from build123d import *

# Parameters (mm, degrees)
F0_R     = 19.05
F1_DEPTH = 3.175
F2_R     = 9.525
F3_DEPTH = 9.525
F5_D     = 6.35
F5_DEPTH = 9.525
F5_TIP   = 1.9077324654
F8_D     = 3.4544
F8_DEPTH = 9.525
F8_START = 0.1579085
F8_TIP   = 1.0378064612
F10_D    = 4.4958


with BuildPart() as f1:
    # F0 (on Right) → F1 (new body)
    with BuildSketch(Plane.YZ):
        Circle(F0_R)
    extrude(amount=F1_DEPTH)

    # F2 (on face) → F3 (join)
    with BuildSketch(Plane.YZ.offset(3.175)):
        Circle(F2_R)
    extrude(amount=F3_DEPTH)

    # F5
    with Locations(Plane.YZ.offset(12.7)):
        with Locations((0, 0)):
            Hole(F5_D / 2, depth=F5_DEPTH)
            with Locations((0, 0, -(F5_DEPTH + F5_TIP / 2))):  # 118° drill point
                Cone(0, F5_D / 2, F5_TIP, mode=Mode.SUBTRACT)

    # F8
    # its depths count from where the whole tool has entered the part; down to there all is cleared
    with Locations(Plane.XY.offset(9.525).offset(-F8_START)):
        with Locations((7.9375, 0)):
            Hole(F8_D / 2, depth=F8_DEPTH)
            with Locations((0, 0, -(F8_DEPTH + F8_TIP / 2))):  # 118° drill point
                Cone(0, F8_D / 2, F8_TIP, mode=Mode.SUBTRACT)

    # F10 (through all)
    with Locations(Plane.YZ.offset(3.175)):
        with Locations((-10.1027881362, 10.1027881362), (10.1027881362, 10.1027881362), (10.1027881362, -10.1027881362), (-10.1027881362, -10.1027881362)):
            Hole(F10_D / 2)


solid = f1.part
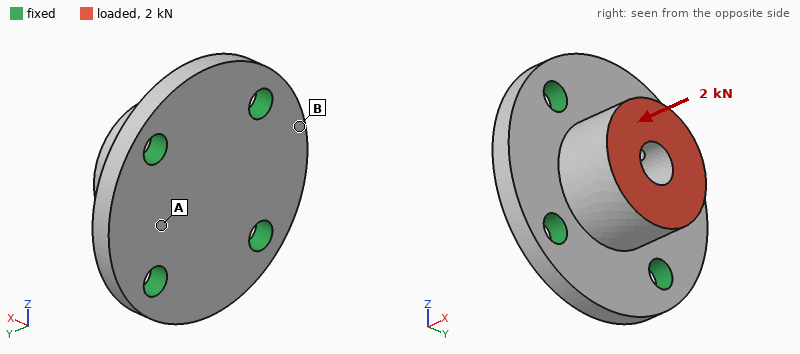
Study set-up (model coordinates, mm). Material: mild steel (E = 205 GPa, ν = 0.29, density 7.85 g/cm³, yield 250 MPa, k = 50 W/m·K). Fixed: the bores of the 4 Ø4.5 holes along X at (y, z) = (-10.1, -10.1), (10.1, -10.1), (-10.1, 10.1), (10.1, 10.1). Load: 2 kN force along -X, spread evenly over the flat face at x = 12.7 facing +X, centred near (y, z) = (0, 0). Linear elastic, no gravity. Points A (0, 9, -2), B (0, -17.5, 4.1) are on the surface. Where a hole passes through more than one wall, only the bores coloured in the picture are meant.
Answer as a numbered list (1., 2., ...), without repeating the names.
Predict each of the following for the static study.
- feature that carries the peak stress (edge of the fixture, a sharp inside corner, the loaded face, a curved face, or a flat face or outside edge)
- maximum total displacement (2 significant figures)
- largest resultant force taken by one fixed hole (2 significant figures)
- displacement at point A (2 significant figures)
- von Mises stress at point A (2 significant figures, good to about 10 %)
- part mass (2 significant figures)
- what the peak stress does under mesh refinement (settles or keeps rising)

1. edge of the fixture
2. 2.5 µm
3. 530 N
4. 1.8 µm
5. 18 MPa
6. 45 g
7. keeps rising
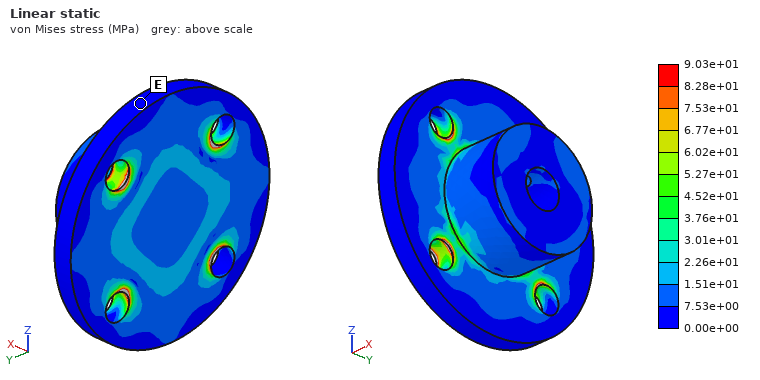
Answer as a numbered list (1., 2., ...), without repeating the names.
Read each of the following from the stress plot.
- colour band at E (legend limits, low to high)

1. 0.00e+00 to 7.53e+00 MPa
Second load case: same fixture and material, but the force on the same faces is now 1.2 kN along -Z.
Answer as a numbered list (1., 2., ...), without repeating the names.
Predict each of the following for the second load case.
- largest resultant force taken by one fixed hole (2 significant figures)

1. 500 N
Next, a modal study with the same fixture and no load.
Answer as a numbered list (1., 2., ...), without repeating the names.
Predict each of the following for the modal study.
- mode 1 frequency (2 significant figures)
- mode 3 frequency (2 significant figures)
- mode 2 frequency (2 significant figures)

1. 28 kHz
2. 29 kHz
3. 28 kHz
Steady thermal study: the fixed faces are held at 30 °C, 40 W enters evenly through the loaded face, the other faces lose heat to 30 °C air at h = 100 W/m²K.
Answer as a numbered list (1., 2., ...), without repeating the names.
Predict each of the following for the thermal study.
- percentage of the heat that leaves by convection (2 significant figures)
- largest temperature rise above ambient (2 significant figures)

1. 14 %
2. 58 K
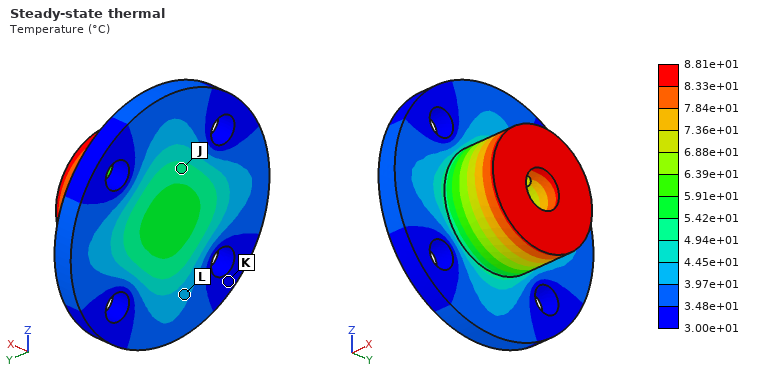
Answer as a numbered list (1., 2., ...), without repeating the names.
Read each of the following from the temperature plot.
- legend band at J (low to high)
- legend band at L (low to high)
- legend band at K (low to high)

1. 4.94e+01 to 5.42e+01 °C
2. 3.97e+01 to 4.45e+01 °C
3. 3.00e+01 to 3.48e+01 °C
